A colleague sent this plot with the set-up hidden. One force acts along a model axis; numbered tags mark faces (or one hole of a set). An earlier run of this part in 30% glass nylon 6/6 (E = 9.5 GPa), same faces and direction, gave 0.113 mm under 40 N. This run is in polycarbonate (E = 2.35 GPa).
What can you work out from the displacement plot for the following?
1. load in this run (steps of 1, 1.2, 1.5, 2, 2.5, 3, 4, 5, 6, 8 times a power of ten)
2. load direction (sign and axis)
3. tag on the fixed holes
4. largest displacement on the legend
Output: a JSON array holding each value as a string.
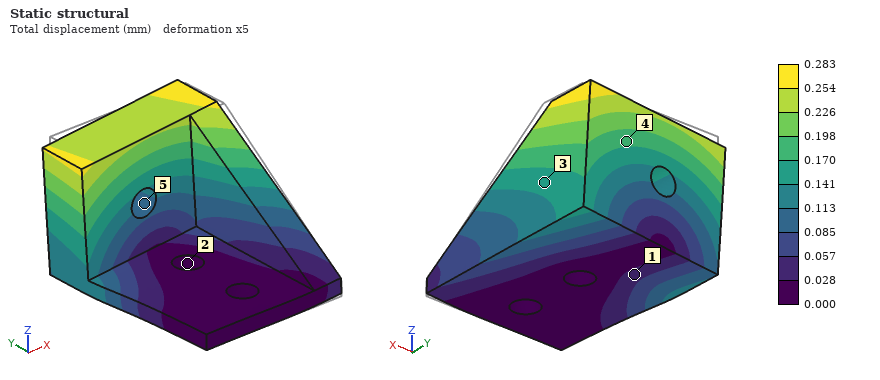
["25 N", "-X", "2", "0.283 mm"]
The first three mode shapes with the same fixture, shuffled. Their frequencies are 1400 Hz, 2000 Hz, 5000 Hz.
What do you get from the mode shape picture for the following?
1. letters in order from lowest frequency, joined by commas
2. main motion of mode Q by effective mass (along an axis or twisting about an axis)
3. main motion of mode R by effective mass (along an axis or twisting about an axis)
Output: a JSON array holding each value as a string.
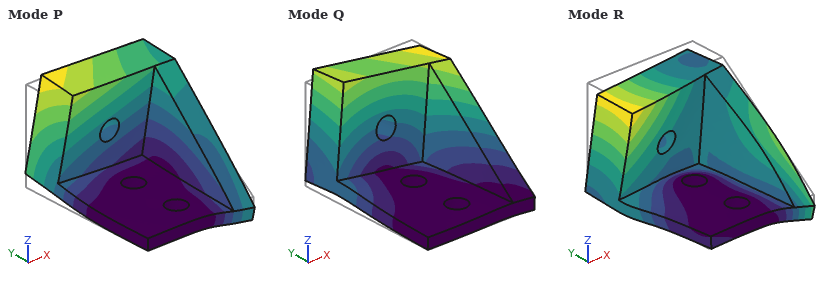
["Q, P, R", "along X", "along Z"]
